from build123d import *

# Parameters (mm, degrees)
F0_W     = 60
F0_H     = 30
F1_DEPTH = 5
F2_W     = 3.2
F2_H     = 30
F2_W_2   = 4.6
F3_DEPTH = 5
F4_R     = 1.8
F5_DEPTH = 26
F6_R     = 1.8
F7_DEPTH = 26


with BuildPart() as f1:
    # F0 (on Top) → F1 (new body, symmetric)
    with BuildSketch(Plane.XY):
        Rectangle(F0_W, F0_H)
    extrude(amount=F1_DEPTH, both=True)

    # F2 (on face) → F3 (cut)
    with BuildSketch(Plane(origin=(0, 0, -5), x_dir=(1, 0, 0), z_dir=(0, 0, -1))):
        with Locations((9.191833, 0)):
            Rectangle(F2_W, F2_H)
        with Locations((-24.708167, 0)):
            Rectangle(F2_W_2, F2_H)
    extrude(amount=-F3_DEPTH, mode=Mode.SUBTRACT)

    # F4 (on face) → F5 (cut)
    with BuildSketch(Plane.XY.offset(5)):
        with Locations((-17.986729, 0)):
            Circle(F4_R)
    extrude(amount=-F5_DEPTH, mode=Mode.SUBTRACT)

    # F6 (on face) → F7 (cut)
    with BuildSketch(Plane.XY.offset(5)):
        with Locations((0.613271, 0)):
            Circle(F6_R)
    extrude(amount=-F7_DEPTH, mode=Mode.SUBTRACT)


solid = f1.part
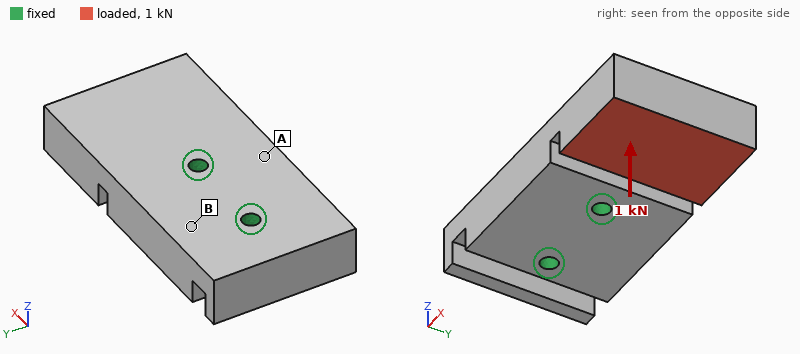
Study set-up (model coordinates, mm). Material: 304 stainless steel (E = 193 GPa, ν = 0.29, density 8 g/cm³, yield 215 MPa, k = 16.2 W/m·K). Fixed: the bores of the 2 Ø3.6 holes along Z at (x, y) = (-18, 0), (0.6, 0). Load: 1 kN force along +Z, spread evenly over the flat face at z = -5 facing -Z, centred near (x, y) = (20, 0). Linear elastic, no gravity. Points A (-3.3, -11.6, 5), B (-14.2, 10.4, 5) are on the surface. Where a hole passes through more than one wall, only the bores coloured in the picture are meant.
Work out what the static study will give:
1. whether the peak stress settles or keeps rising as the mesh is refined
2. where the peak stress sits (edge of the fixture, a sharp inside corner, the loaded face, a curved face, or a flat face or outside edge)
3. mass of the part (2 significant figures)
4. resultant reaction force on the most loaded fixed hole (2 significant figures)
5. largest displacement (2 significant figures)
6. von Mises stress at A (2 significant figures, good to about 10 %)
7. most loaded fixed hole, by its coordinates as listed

keeps rising
edge of the fixture
130 g
1.4 kN
40 µm
17 MPa
(0.6, 0)
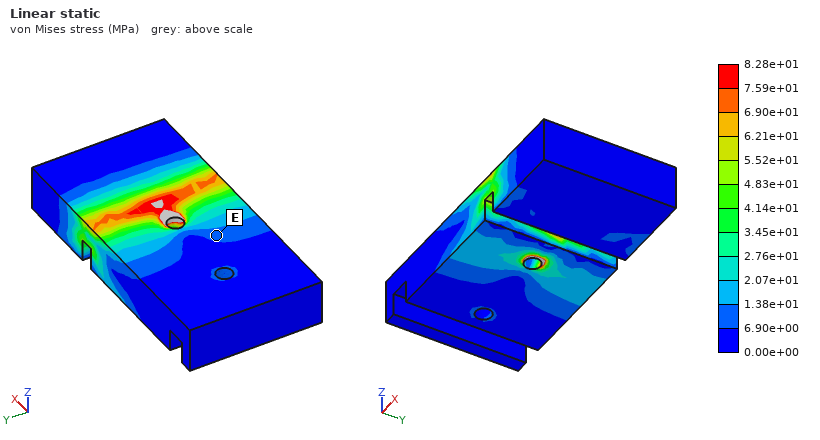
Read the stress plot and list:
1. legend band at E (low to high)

6.90e+00 to 1.38e+01 MPa
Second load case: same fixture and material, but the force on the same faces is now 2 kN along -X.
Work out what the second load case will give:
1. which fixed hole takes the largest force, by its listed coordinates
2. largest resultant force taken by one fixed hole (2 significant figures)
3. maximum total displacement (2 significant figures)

(0.6, 0)
1.5 kN
45 µm
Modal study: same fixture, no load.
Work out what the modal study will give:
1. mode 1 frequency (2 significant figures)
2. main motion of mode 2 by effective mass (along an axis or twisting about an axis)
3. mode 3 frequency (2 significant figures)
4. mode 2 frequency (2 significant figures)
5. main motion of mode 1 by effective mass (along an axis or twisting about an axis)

4400 Hz
along Y
11 kHz
9800 Hz
along Z
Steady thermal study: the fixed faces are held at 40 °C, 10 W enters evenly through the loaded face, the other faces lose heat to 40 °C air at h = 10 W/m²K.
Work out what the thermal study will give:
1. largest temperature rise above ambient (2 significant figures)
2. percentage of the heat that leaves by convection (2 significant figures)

64 K
10 %
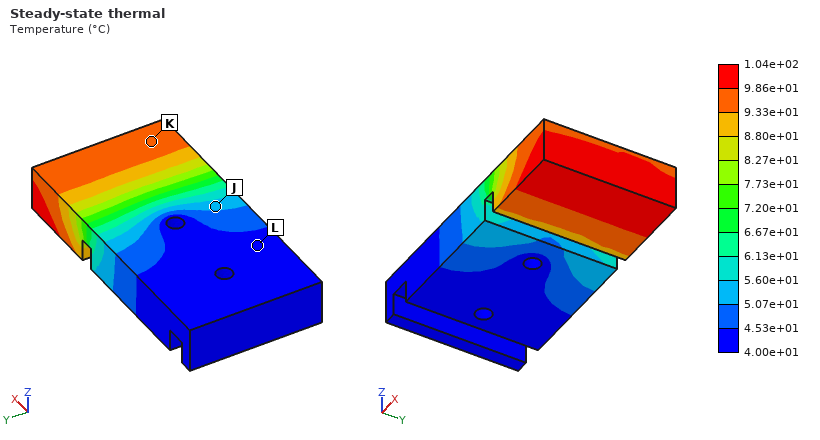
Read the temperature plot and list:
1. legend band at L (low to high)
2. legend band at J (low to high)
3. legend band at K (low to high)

4.00e+01 to 4.53e+01 °C
5.07e+01 to 5.60e+01 °C
9.33e+01 to 9.86e+01 °C
